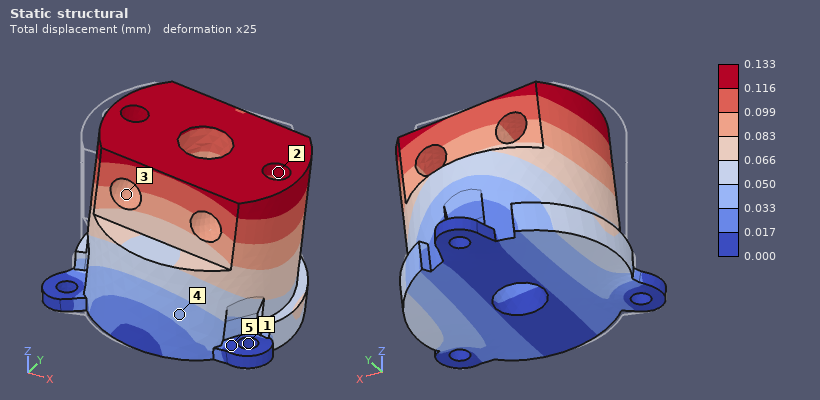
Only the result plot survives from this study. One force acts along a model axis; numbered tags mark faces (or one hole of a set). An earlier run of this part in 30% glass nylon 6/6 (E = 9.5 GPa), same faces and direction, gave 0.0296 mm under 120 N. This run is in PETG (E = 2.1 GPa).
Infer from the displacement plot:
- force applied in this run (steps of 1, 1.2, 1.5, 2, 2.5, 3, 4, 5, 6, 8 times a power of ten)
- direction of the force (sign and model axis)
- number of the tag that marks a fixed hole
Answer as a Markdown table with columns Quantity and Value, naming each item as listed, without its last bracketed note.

| Quantity | Value |
|---|---|
| force applied in this run | 120 N |
| direction of the force | +X |
| number of the tag that marks a fixed hole | 1 |
